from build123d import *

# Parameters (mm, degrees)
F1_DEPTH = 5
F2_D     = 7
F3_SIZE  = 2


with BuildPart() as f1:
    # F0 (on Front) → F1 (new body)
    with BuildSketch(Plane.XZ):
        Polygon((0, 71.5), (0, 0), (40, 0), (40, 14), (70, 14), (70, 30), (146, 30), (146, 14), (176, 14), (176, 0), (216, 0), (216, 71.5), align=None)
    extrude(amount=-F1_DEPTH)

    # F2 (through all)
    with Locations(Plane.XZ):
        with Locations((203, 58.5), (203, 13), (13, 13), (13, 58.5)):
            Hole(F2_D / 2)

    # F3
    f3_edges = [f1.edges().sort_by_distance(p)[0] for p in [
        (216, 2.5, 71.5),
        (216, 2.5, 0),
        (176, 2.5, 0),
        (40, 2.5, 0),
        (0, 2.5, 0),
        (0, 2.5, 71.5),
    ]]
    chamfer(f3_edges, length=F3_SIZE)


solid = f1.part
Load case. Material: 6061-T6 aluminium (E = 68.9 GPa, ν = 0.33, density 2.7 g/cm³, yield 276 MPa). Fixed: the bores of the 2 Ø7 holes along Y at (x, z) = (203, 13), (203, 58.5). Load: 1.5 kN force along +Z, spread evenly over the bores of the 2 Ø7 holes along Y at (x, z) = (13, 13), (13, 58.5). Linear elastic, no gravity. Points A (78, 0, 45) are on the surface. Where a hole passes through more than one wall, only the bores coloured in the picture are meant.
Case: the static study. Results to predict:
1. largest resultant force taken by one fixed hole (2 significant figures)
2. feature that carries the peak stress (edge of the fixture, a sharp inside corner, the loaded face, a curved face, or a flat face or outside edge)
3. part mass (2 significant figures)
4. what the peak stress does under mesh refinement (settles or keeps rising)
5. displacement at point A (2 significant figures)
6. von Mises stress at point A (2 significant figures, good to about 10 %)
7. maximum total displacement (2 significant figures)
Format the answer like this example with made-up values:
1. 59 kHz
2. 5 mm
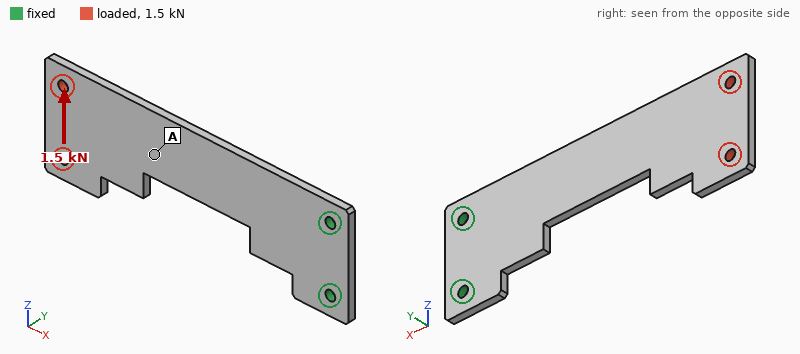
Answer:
1. 6.1 kN
2. a sharp inside corner
3. 160 g
4. keeps rising
5. 0.50 mm
6. 23 MPa
7. 1.3 mm
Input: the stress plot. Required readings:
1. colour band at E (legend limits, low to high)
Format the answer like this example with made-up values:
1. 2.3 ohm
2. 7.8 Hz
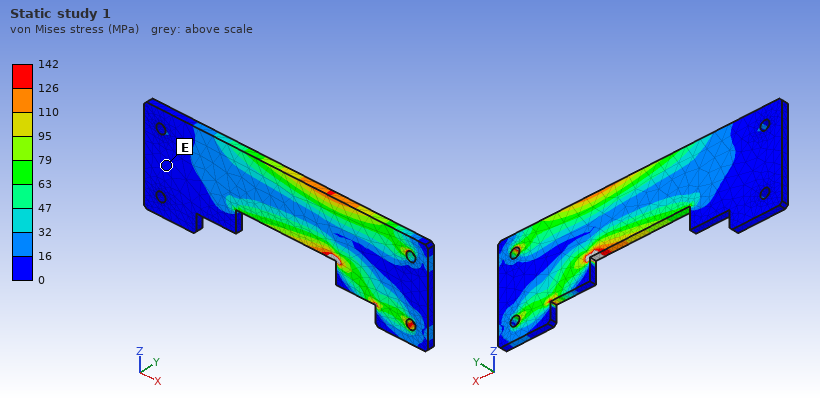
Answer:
1. 0 to 16 MPa
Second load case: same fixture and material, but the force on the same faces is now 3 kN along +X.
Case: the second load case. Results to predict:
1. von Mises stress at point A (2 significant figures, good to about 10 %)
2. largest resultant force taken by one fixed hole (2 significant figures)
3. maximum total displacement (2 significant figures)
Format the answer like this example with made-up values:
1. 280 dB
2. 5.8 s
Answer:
1. 19 MPa
2. 1.6 kN
3. 0.31 mm
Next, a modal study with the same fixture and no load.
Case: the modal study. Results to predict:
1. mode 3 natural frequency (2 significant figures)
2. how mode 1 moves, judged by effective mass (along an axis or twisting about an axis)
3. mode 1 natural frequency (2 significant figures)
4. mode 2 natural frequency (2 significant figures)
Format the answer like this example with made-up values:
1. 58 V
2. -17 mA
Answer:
1. 670 Hz
2. along Y
3. 92 Hz
4. 520 Hz
